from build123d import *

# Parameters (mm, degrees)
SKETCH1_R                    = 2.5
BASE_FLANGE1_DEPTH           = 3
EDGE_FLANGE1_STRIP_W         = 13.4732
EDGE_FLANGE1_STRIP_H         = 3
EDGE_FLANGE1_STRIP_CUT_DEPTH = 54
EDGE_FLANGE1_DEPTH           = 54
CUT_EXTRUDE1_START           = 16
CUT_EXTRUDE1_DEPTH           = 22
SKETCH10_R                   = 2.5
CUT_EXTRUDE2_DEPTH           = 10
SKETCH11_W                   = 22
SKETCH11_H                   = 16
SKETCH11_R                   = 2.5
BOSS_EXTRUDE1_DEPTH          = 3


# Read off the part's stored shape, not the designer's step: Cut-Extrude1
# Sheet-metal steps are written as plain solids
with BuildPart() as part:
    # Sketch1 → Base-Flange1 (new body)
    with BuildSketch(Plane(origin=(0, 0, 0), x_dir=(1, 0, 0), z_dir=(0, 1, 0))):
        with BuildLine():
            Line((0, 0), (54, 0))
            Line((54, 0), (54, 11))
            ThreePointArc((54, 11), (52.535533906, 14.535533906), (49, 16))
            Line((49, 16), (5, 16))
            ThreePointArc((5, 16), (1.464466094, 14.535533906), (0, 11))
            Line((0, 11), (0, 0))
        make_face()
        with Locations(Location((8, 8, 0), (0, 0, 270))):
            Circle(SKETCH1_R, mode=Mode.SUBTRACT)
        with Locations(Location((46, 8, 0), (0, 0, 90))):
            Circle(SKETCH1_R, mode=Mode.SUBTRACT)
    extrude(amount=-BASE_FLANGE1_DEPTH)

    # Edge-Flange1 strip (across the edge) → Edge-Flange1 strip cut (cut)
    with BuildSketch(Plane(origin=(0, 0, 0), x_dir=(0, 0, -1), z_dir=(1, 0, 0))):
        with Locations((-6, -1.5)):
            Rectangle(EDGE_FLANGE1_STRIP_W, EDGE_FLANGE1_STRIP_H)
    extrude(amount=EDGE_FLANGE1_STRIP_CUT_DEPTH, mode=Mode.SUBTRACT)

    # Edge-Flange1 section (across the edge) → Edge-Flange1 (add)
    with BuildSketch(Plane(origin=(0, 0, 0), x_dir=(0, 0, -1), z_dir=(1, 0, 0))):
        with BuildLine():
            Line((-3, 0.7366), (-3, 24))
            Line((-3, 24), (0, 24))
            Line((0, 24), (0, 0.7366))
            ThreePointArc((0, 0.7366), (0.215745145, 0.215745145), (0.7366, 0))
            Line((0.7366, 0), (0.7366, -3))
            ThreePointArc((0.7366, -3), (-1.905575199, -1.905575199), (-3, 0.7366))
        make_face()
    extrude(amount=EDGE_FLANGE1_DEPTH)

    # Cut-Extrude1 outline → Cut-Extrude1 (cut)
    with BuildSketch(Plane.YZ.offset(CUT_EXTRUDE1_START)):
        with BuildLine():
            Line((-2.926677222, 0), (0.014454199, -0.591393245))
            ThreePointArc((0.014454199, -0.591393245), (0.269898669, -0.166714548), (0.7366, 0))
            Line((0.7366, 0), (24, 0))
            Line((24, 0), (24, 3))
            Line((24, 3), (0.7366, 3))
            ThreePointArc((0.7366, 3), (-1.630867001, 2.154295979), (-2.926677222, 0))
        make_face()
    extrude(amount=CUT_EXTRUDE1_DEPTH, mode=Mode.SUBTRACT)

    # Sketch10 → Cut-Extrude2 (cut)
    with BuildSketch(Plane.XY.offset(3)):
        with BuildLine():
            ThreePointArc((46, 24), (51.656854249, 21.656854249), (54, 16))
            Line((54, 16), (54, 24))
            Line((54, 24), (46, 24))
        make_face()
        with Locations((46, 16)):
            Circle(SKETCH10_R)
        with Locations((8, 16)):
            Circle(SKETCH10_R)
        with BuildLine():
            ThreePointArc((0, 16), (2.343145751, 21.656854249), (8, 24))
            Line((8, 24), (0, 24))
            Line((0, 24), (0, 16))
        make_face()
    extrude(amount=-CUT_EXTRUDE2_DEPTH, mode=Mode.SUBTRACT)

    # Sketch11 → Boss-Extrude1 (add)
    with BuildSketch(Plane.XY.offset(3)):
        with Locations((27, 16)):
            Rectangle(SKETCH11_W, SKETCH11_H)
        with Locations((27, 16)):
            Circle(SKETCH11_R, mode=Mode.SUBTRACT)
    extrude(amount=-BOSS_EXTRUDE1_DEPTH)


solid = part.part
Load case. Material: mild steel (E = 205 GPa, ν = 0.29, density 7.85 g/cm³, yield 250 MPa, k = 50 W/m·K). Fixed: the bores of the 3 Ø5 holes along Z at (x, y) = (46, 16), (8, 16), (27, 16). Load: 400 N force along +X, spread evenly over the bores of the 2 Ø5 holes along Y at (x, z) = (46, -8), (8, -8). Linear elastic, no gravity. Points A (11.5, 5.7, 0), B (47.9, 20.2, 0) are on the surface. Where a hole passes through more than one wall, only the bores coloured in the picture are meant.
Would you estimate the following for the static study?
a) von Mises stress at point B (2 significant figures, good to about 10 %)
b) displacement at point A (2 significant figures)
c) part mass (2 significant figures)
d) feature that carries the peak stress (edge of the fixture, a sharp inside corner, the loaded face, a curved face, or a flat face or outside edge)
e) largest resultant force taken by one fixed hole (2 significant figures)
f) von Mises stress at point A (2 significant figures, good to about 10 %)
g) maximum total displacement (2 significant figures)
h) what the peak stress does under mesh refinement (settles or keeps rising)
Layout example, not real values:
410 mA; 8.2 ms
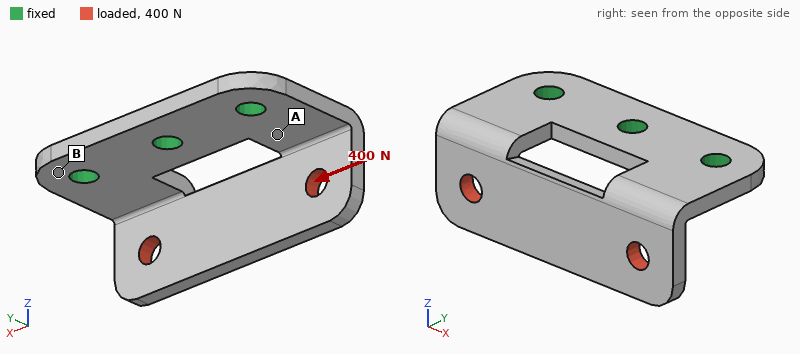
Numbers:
6.2 MPa; 3.5 µm; 45 g; a sharp inside corner; 200 N; 28 MPa; 19 µm; keeps rising
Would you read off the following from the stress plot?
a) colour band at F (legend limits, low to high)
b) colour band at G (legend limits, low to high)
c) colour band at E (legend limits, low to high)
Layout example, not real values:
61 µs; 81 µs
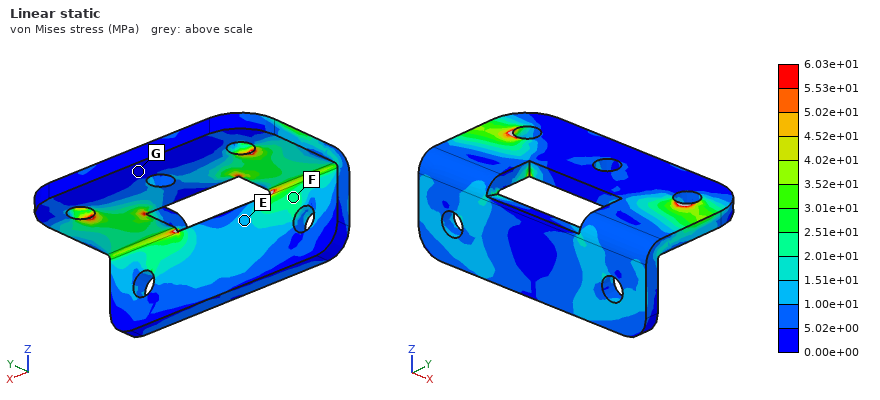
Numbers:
2.01e+01 to 2.51e+01 MPa; 0.00e+00 to 5.02e+00 MPa; 1.00e+01 to 1.51e+01 MPa
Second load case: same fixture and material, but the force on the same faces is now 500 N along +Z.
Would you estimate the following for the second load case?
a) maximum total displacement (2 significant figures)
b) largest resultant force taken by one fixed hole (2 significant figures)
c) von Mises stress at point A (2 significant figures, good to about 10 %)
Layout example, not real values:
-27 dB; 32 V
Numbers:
86 µm; 240 N; 73 MPa
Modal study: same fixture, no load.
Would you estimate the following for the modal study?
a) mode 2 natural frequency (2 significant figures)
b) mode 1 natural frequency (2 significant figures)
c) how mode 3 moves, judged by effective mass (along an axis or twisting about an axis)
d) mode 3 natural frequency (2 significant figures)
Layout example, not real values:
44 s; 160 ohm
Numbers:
4400 Hz; 2500 Hz; along Z; 6600 Hz
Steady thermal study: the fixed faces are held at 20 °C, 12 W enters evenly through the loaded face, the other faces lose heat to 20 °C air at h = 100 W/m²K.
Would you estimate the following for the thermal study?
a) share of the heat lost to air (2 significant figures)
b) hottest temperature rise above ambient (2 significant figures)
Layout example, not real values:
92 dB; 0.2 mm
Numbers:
54 %; 37 K
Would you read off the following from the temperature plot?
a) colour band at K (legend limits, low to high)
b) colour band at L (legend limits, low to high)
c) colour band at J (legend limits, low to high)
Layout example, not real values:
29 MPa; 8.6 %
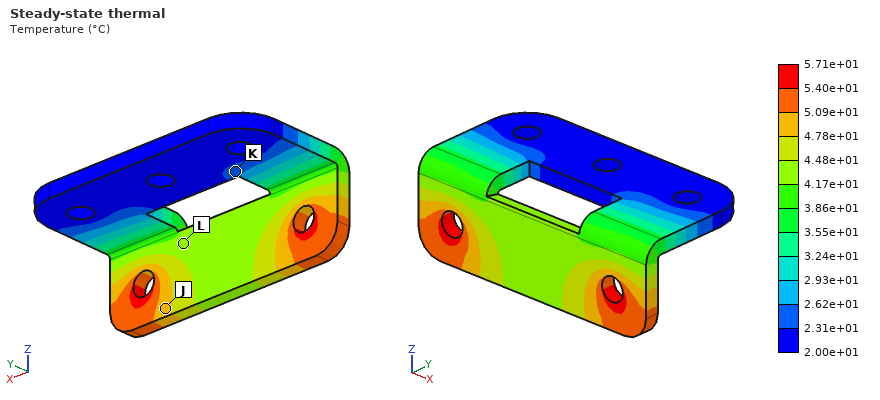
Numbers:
2.31e+01 to 2.62e+01 °C; 4.17e+01 to 4.48e+01 °C; 4.78e+01 to 5.09e+01 °C
